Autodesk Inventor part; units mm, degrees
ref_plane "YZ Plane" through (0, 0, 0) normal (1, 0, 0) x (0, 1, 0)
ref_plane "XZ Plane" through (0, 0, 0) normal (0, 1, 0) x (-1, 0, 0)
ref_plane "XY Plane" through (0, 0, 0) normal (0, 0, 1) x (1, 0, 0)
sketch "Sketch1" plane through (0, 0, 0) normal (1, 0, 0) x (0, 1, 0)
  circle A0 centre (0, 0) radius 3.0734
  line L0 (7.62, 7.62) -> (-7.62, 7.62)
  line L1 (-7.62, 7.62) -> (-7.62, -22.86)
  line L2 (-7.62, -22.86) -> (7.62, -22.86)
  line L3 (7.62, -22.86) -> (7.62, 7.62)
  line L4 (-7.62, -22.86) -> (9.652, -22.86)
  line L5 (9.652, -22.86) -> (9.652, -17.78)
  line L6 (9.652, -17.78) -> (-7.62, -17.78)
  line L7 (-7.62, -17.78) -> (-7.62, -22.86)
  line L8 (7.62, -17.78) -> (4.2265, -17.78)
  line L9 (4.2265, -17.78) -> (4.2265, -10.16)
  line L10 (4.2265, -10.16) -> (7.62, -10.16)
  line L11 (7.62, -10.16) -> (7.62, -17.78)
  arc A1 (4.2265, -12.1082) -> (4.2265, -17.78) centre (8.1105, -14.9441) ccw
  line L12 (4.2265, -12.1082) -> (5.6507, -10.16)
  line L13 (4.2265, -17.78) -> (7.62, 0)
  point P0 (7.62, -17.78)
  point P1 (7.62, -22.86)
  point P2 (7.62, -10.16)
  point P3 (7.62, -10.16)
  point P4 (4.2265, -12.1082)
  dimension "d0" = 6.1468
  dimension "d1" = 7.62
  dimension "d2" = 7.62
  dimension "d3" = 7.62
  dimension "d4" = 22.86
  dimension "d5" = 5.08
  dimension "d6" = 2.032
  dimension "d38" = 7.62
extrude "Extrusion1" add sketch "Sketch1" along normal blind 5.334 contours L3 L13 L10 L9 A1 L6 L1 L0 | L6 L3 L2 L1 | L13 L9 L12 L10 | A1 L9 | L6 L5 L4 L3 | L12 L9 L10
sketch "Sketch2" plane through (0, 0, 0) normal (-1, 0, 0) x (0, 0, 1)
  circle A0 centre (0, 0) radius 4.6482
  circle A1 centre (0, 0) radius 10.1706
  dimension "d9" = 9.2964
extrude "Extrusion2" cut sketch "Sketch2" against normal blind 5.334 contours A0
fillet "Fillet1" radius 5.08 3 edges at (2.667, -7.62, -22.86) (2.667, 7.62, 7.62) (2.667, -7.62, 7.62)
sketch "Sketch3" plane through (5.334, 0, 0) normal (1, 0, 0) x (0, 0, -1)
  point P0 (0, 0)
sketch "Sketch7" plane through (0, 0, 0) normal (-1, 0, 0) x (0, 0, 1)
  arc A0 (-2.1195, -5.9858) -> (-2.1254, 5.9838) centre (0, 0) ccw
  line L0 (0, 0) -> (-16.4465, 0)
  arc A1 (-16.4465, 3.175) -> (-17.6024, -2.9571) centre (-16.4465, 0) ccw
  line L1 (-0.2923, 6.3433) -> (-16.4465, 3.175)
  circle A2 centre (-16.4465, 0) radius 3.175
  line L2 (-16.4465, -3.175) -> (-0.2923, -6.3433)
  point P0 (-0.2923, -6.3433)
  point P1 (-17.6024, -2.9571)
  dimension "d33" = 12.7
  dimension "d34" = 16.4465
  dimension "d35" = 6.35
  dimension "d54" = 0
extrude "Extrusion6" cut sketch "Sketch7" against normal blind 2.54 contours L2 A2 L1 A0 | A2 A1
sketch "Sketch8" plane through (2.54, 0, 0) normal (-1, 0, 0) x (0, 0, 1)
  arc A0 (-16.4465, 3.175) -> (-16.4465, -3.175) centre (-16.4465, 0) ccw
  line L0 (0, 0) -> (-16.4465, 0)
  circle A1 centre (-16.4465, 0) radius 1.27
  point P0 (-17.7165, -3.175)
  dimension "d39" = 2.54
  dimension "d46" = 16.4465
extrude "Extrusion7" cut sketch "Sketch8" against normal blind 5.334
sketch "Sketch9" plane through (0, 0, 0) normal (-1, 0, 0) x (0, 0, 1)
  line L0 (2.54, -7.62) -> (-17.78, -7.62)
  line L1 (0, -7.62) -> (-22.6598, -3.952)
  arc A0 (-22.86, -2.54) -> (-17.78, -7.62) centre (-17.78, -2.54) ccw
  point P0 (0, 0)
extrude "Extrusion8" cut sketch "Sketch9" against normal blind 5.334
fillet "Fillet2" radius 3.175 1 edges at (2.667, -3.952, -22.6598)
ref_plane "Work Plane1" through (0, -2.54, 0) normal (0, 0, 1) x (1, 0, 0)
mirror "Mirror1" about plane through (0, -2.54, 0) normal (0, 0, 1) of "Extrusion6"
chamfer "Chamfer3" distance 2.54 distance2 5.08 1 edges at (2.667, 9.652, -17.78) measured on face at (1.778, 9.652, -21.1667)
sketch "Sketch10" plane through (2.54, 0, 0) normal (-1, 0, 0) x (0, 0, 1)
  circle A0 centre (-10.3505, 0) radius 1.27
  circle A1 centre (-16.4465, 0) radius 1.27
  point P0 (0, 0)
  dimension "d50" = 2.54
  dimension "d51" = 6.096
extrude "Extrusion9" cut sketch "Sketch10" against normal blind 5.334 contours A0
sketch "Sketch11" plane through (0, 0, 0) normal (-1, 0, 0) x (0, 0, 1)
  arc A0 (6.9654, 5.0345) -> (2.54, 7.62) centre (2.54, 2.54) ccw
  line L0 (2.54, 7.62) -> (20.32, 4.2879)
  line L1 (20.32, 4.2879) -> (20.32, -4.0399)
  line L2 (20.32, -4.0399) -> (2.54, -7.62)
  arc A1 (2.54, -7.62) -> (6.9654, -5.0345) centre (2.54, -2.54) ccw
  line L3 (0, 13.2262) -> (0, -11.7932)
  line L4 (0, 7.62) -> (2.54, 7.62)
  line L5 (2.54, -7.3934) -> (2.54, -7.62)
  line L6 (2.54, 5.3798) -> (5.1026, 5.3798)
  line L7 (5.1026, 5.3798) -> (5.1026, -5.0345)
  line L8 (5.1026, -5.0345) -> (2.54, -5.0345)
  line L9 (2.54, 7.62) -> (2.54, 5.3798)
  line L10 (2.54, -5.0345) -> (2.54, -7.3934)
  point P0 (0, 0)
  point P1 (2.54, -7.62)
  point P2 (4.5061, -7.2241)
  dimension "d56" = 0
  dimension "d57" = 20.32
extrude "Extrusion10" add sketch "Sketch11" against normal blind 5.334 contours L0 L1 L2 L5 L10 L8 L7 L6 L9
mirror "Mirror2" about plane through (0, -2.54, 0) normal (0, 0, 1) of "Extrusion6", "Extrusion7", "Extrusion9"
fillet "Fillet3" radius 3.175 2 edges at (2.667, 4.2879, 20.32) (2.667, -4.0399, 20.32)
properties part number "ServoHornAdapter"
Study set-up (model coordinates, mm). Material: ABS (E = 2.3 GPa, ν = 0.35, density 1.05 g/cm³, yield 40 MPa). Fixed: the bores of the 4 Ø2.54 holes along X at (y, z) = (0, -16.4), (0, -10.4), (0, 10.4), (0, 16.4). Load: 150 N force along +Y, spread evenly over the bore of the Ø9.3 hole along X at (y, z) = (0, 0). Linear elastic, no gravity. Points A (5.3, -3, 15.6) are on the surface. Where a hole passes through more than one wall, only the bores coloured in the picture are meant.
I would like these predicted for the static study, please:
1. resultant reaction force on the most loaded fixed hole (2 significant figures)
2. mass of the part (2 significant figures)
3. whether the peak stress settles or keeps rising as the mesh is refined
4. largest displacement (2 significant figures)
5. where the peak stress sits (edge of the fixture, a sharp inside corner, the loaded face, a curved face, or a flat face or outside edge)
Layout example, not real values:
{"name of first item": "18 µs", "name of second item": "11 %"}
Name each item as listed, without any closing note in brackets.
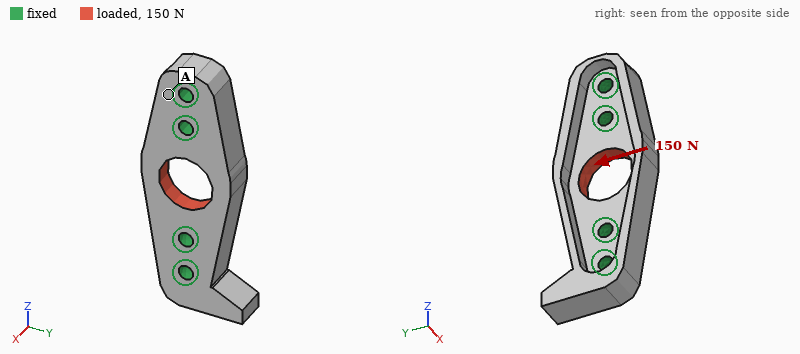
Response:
{"resultant reaction force on the most loaded fixed hole": "85 N", "mass of the part": "1.8 g", "whether the peak stress settles or keeps rising as the mesh is refined": "keeps rising", "largest displacement": "33 µm", "where the peak stress sits": "edge of the fixture"}
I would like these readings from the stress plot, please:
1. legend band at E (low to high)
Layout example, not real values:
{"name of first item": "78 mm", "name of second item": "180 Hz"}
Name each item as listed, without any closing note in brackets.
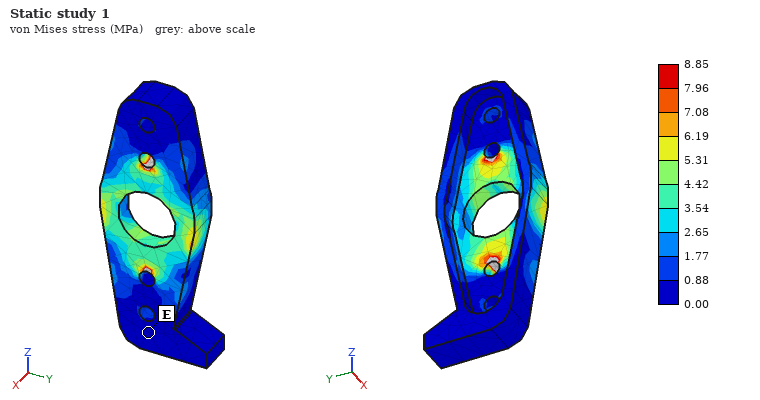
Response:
{"legend band at E": "0.00 to 0.88 MPa"}
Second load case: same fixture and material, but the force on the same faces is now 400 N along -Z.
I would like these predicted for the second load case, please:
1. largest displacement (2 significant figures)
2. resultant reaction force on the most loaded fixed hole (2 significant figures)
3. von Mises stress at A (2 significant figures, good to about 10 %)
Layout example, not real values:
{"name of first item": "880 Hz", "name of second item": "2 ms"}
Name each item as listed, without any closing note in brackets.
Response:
{"largest displacement": "34 µm", "resultant reaction force on the most loaded fixed hole": "150 N", "von Mises stress at A": "1.9 MPa"}
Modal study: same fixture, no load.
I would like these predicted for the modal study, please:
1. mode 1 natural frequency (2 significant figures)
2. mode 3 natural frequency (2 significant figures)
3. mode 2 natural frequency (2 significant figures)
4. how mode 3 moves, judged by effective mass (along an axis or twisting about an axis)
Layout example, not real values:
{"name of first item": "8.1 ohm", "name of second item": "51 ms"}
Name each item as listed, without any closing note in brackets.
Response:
{"mode 1 natural frequency": "7200 Hz", "mode 3 natural frequency": "8300 Hz", "mode 2 natural frequency": "7300 Hz", "how mode 3 moves, judged by effective mass": "along X"}
